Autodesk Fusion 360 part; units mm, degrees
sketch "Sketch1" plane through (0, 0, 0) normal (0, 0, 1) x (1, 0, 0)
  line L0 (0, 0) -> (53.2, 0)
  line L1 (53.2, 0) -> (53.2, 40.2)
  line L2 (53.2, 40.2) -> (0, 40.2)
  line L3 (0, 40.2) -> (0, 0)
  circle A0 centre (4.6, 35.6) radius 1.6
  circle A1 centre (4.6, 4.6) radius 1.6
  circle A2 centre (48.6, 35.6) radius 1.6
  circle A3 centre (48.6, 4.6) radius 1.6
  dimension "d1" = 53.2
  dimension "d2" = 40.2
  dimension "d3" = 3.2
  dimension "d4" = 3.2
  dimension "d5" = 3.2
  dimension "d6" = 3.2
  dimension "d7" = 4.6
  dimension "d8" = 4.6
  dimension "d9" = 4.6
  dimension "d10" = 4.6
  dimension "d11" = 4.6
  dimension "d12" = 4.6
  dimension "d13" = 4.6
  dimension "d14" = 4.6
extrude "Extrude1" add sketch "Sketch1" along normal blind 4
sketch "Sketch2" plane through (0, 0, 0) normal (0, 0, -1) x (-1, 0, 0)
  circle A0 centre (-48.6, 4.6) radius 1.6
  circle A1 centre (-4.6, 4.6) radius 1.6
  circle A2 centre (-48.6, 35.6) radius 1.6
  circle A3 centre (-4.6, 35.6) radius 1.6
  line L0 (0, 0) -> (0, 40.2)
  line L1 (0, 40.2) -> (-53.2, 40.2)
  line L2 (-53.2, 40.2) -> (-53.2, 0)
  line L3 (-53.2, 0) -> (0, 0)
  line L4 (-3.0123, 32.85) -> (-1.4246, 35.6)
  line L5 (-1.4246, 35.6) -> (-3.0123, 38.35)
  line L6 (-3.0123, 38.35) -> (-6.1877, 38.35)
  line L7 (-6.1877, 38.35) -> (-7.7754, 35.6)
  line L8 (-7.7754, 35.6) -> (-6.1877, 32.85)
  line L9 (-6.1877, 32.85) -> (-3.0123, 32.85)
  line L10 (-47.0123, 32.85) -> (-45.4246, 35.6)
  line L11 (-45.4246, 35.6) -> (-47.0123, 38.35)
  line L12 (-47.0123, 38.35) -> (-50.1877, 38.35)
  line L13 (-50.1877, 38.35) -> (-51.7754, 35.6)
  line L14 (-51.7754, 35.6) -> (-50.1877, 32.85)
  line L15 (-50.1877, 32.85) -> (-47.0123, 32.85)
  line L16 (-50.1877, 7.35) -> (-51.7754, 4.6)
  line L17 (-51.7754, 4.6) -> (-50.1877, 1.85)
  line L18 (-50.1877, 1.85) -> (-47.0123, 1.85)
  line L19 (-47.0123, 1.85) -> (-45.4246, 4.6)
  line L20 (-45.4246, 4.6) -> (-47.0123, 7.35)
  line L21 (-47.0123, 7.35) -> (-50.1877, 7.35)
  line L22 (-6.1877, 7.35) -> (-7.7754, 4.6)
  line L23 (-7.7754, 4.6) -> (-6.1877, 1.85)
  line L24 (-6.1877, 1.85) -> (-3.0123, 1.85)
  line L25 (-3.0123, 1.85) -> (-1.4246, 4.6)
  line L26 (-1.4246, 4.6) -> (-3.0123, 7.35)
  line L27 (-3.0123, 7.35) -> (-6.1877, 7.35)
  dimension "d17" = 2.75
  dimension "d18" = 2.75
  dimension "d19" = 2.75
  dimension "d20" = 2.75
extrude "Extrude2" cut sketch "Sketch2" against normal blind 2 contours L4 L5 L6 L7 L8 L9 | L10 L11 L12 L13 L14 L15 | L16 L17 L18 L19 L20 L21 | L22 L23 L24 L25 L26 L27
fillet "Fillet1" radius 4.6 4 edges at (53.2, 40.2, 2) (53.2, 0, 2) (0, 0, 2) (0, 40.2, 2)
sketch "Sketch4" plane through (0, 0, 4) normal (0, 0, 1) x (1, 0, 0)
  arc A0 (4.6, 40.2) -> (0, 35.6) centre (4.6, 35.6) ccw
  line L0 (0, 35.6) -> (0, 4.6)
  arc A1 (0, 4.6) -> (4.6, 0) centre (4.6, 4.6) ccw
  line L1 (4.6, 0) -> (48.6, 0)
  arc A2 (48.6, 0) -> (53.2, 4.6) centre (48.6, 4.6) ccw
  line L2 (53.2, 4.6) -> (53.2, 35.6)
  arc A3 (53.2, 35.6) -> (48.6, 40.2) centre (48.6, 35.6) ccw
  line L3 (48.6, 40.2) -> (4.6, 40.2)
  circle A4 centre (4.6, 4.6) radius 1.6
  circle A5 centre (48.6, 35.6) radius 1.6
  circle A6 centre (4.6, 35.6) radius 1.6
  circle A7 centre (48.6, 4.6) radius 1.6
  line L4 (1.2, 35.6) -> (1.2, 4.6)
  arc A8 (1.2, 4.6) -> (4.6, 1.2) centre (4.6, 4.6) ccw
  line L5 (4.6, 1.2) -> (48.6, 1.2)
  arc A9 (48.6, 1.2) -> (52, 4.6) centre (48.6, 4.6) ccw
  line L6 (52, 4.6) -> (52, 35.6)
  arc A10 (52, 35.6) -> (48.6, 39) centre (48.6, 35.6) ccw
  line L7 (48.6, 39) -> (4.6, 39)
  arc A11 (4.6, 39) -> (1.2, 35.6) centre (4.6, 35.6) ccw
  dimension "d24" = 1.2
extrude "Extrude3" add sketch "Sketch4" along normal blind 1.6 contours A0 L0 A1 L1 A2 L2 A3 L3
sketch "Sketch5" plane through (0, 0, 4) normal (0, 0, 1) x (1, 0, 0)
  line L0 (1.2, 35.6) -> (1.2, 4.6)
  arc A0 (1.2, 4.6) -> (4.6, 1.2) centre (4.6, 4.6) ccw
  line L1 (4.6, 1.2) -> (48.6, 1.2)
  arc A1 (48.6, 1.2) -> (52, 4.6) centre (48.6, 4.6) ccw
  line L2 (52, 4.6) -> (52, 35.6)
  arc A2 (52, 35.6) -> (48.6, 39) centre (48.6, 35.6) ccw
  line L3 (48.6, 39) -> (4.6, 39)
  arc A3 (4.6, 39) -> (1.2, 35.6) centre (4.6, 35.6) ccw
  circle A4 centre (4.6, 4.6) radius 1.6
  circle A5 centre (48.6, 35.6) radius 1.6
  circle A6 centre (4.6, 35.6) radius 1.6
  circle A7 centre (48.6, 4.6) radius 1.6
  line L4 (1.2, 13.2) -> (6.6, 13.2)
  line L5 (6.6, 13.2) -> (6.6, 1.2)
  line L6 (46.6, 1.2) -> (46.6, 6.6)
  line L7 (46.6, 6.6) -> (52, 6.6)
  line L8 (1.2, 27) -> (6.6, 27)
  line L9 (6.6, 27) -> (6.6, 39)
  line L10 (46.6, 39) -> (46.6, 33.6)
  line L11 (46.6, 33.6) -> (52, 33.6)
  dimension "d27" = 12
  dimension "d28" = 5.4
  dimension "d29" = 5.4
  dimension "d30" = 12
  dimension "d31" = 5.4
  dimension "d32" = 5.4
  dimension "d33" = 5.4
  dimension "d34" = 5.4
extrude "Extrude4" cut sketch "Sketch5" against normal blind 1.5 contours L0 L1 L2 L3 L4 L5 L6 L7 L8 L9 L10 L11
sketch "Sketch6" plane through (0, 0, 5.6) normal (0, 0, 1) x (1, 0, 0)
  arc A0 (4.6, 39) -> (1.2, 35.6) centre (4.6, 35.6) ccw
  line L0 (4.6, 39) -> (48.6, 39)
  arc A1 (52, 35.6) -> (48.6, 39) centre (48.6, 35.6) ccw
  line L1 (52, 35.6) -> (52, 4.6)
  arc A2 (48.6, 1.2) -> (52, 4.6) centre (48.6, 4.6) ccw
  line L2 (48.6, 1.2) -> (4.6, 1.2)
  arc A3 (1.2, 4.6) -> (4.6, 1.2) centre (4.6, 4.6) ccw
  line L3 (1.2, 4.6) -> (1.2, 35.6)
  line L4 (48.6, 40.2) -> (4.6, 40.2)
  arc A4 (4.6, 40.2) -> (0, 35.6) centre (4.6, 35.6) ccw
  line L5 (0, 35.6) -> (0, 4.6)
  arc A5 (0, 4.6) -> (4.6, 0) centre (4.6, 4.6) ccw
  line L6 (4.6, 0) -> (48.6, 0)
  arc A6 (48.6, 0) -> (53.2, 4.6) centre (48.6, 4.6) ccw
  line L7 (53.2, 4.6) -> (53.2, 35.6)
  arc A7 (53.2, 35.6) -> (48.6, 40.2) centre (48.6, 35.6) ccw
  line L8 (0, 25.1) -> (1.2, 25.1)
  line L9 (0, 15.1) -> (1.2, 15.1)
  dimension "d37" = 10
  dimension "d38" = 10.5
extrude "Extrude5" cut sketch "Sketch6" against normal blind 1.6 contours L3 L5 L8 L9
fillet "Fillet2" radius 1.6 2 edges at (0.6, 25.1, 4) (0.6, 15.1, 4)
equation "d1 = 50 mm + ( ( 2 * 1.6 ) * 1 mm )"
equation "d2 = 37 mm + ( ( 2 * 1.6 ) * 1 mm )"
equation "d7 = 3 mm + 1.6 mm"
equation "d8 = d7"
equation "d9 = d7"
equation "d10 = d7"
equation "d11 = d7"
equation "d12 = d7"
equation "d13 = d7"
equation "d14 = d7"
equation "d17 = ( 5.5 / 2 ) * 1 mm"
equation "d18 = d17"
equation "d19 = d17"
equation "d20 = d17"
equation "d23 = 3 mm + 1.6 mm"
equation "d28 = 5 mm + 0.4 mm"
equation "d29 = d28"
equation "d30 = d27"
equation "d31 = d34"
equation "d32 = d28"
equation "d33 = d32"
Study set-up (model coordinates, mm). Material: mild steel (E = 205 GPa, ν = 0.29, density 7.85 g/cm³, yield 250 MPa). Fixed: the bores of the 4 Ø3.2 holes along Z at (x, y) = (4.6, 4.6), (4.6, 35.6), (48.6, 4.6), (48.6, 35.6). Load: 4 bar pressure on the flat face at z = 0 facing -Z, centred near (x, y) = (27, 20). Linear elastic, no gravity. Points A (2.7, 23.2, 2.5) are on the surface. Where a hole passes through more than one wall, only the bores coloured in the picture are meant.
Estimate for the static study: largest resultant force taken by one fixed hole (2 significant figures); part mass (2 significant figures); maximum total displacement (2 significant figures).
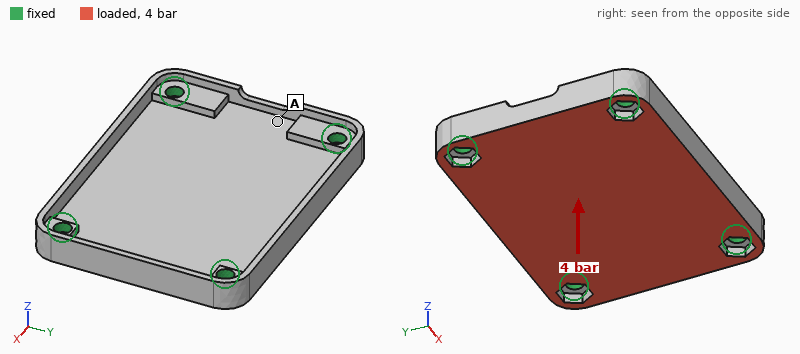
370 N
47 g
20 µm
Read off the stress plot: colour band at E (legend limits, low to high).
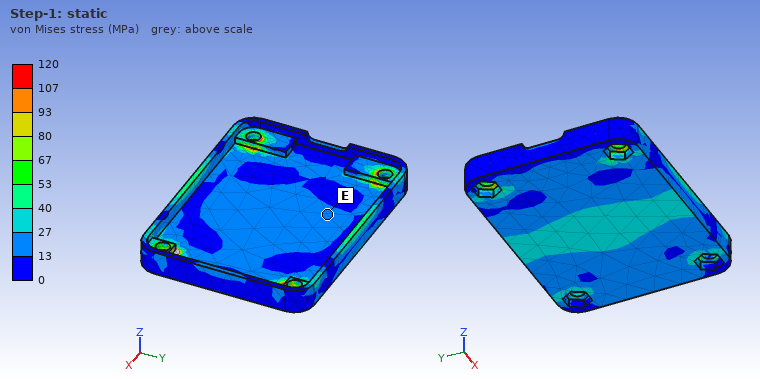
13 to 27 MPa
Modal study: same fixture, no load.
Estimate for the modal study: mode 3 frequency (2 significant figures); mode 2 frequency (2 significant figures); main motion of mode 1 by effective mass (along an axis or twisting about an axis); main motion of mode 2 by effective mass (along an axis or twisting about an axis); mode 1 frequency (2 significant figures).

12 kHz
8900 Hz
along Z
twisting about X
6100 Hz
